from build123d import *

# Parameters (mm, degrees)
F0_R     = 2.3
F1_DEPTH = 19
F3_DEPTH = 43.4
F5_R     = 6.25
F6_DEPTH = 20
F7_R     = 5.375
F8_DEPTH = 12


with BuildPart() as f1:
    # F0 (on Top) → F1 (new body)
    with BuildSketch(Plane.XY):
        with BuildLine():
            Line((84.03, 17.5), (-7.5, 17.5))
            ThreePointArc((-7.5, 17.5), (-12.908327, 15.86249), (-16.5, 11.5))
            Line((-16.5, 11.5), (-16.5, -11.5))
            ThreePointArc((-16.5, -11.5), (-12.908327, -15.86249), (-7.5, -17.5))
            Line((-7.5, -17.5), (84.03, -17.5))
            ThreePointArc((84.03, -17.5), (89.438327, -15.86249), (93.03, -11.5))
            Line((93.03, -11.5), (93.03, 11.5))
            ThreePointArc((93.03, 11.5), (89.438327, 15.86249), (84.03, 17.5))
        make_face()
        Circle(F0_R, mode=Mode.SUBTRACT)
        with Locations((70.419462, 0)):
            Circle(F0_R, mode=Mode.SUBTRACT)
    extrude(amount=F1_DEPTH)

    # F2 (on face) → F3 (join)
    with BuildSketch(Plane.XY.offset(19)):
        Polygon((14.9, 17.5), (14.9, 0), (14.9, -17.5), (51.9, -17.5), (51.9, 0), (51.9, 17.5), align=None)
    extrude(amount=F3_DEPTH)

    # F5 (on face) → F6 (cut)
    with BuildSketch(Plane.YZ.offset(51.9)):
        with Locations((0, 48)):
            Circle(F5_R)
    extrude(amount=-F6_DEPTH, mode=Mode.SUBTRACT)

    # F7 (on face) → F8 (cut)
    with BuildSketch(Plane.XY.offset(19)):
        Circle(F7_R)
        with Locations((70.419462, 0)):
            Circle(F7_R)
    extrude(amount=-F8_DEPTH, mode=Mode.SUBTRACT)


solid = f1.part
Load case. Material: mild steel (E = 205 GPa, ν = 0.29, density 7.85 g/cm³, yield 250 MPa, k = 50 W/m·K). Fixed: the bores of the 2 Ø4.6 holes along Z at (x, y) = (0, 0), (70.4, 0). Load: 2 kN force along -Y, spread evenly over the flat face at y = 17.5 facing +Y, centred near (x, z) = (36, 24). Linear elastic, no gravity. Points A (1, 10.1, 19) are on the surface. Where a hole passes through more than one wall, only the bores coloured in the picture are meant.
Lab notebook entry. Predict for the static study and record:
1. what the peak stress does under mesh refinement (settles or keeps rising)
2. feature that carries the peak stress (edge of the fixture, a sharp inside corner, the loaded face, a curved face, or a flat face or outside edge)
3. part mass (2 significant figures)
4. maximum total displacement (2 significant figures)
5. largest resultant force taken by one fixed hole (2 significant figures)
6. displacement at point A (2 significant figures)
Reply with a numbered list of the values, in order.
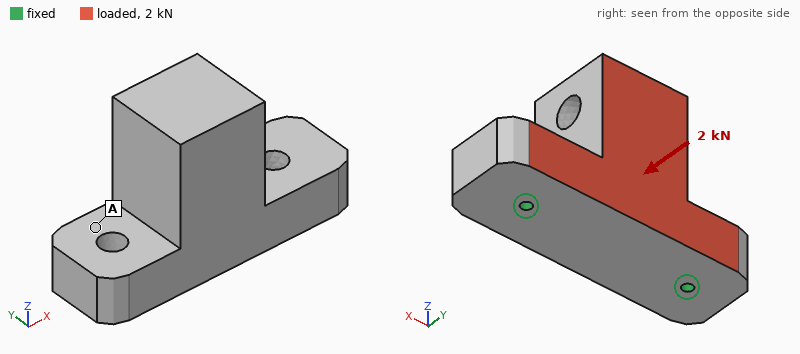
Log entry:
1. keeps rising
2. edge of the fixture
3. 970 g
4. 37 µm
5. 1.0 kN
6. 10 µm
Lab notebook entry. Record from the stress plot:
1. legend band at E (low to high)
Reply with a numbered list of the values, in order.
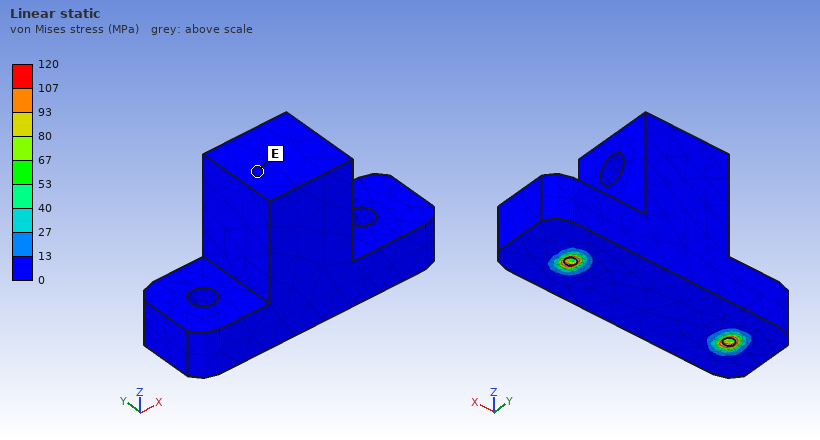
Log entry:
1. 0 to 13 MPa
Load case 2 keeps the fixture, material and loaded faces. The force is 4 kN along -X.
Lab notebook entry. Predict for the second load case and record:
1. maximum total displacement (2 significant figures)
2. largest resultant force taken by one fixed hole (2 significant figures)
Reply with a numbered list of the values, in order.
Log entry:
1. 6.0 µm
2. 2.6 kN
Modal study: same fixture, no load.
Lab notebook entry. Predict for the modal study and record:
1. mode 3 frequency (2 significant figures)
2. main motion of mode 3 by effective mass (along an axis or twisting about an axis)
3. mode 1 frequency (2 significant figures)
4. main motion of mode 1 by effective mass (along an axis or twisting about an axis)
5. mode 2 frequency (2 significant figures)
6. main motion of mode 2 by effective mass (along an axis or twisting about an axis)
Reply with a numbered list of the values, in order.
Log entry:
1. 6600 Hz
2. along Z
3. 1500 Hz
4. along Y
5. 6000 Hz
6. along X
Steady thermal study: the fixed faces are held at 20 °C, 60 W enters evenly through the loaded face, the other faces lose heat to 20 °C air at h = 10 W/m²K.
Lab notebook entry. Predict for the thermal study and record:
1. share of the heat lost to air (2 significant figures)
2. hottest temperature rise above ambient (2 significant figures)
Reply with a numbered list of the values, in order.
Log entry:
1. 7.9 %
2. 47 K
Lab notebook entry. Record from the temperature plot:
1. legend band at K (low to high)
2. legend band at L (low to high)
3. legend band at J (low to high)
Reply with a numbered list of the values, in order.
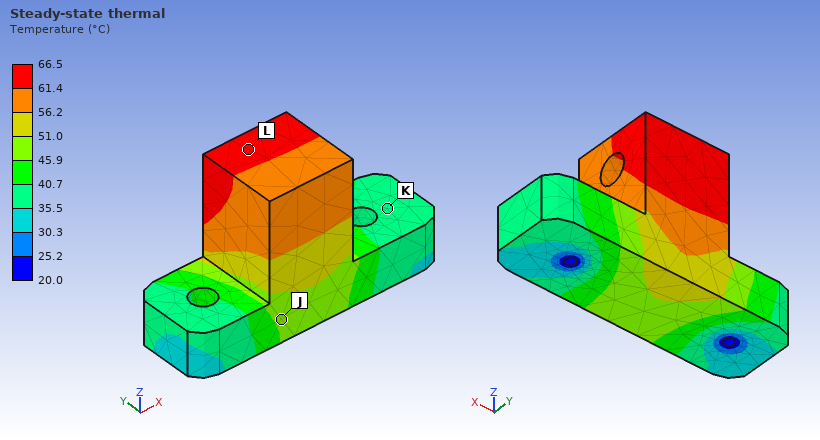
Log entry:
1. 35.5 to 40.7 °C
2. 61.4 to 66.5 °C
3. 45.9 to 51.0 °C
